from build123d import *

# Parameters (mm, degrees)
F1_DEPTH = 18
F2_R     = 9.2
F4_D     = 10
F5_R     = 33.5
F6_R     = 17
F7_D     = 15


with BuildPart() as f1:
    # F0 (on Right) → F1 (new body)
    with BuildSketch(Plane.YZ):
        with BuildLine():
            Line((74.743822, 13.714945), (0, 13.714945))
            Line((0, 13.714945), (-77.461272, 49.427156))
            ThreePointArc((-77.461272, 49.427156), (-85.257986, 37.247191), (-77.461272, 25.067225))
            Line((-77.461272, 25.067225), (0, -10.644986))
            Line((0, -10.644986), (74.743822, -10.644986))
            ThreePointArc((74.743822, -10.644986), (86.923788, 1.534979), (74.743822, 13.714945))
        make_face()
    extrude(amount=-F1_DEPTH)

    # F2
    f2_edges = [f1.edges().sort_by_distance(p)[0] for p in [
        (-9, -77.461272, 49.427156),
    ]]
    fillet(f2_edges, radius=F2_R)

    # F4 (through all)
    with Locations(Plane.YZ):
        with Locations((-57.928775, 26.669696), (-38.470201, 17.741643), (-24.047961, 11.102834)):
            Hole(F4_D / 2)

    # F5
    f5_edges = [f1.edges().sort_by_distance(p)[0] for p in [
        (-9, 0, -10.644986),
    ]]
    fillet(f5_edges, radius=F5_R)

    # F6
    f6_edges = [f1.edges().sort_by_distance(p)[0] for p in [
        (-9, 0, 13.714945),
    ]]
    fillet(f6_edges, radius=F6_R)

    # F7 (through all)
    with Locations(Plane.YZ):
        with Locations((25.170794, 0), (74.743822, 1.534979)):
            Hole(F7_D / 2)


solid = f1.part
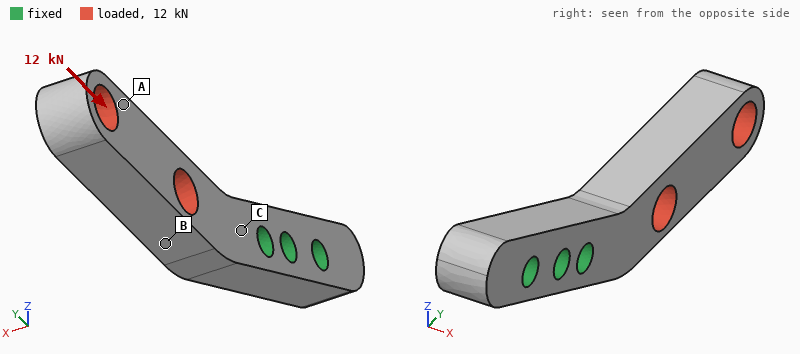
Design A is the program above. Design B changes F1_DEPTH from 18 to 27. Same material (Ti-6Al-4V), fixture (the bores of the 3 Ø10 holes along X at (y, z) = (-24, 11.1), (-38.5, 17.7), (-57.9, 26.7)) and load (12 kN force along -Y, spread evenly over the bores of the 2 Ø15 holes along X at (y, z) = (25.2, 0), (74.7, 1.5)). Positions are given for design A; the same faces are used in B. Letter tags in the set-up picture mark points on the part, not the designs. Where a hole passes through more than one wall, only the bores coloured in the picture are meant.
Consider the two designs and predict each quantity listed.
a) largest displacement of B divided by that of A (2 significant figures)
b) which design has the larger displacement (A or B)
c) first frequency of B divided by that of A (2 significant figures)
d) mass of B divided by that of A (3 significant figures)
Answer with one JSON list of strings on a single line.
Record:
["0.66", "A", "1.2", "1.50"]
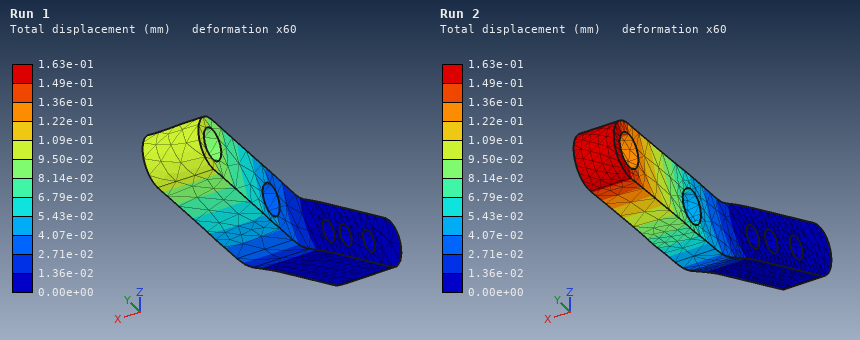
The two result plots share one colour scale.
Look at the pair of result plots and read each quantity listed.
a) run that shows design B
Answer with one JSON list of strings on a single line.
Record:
["Run 1"]
